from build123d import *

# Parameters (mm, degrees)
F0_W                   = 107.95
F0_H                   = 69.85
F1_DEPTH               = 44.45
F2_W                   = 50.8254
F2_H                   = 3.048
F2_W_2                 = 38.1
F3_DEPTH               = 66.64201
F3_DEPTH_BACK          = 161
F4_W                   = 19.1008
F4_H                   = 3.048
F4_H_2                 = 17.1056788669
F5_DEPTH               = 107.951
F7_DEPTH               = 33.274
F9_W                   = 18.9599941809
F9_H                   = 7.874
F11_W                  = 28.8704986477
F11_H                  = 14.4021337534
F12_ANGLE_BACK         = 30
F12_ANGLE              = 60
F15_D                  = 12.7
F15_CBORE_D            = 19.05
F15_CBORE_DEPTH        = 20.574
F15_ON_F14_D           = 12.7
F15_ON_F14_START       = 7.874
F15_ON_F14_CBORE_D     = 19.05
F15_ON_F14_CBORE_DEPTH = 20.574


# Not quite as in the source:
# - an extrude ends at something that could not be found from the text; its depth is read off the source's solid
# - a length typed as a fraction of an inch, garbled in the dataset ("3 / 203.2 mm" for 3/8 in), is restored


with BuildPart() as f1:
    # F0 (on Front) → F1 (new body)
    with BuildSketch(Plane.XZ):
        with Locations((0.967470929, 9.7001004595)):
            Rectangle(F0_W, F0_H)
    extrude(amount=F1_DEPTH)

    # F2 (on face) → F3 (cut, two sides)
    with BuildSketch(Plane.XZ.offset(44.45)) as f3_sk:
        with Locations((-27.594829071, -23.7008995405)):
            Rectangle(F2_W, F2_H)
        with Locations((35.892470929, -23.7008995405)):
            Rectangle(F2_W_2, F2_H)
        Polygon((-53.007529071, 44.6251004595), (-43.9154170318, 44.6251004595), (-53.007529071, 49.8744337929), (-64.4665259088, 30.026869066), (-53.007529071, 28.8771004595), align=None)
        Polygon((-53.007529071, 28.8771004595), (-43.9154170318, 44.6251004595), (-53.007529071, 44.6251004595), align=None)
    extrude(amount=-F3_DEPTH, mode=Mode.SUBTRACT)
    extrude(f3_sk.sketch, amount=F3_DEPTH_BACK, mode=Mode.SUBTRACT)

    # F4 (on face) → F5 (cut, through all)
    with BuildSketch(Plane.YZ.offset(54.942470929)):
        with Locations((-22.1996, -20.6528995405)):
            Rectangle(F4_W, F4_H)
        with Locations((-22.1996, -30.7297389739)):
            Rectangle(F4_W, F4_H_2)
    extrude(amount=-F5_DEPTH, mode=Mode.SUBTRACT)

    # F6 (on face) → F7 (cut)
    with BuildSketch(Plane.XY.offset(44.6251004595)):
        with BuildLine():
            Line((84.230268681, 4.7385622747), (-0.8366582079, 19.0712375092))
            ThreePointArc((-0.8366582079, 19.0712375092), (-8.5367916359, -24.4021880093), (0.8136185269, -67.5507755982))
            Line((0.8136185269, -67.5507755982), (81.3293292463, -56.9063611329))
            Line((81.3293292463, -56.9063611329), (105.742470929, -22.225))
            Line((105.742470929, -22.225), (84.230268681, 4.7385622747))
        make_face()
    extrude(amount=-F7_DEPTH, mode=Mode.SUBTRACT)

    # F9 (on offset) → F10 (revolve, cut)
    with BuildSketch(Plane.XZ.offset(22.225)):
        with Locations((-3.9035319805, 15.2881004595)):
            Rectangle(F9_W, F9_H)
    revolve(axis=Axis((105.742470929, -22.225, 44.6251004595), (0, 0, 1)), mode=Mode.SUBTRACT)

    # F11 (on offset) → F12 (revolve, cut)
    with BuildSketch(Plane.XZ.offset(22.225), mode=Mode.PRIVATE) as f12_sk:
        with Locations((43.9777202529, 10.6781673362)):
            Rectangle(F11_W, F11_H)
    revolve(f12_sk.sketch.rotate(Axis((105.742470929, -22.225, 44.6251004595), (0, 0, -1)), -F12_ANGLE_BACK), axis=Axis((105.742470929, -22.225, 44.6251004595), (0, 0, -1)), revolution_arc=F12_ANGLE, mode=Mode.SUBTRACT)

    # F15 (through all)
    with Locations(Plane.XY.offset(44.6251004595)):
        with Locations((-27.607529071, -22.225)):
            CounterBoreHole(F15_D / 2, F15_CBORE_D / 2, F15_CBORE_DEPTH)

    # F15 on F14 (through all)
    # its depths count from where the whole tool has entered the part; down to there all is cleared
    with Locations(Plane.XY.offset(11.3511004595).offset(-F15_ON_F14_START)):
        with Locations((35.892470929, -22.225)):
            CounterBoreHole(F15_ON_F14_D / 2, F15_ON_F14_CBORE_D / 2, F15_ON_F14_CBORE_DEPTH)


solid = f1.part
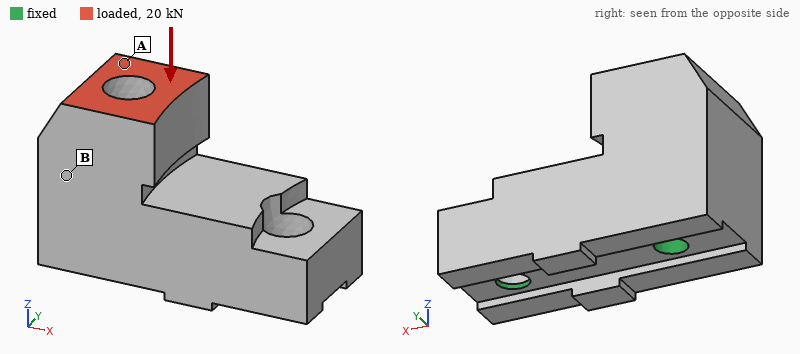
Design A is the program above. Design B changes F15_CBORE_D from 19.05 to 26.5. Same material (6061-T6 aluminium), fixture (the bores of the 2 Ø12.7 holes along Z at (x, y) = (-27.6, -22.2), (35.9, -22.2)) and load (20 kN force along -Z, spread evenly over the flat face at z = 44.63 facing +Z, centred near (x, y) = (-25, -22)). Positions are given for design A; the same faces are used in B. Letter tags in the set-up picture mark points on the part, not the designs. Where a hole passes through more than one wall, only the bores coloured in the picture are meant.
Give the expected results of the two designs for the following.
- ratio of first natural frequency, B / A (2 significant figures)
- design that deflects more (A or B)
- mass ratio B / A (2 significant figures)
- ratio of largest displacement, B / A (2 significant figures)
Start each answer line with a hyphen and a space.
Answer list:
- 1.00
- B
- 0.97
- 1.3
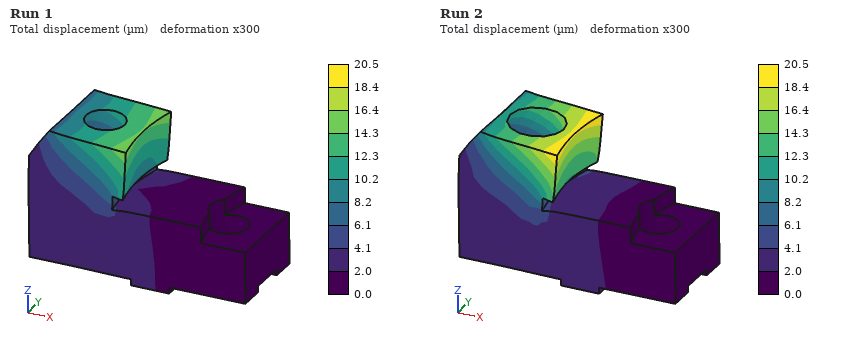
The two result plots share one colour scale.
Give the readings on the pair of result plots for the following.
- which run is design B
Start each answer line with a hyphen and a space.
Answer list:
- Run 2
